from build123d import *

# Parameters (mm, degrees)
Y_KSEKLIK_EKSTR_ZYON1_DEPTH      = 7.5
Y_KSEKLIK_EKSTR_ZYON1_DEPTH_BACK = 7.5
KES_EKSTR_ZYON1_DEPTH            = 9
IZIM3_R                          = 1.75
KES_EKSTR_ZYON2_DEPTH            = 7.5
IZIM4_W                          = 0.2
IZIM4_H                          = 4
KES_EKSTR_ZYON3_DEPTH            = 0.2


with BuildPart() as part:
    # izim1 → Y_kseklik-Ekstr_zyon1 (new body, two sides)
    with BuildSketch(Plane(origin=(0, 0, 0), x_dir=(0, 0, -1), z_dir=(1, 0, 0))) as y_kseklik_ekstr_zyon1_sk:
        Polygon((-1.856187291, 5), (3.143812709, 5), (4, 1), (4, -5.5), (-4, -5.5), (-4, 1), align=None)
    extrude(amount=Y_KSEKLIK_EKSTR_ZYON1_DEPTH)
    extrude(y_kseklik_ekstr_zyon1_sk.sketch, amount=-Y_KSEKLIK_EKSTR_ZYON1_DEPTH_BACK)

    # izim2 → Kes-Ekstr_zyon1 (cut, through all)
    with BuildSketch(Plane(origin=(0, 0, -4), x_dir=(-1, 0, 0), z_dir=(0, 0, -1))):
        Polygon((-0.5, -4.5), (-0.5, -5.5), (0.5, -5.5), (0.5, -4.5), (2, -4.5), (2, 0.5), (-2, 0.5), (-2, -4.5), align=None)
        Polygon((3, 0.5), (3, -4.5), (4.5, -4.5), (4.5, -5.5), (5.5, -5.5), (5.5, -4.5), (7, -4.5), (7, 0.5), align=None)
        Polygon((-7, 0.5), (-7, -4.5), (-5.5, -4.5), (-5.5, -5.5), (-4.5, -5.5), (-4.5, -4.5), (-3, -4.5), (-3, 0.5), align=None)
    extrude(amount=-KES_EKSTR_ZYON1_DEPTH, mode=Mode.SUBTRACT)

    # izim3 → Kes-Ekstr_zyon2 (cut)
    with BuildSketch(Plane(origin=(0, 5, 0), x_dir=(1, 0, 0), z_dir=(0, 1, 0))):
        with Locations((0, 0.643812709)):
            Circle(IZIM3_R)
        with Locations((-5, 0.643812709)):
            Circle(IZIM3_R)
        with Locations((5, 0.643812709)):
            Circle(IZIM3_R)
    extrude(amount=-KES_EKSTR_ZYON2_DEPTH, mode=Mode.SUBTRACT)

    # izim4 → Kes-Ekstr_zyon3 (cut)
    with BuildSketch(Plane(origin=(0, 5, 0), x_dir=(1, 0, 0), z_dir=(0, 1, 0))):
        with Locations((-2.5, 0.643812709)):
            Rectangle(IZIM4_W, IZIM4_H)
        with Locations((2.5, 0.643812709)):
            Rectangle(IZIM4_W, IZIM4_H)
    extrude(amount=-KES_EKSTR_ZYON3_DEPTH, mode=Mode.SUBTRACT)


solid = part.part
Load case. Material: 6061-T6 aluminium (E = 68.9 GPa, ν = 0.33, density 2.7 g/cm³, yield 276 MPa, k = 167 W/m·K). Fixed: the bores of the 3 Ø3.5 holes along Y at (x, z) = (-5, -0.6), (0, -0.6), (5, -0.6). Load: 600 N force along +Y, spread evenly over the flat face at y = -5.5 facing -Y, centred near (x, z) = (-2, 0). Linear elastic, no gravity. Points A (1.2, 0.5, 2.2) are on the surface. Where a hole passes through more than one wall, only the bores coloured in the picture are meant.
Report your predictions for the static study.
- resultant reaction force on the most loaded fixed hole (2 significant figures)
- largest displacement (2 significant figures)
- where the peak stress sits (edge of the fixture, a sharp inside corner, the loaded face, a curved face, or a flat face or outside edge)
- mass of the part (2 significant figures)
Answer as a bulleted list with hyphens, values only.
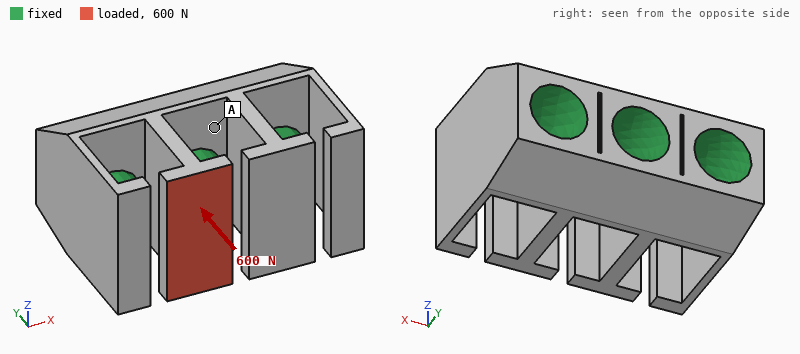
- 320 N
- 12 µm
- the loaded face
- 1.4 g
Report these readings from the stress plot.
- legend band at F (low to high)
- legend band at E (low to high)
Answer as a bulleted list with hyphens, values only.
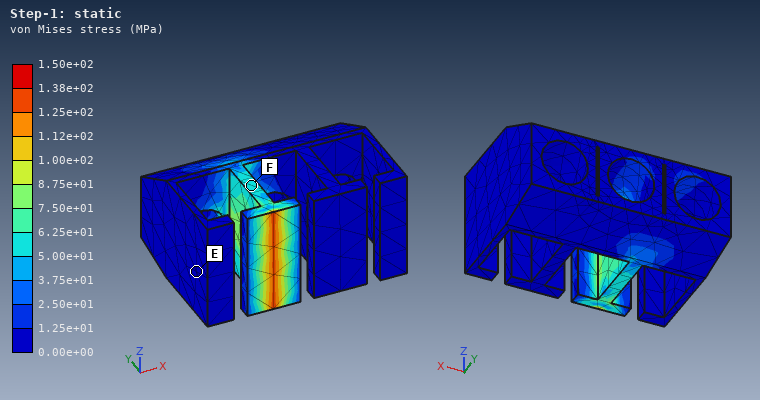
- 5.00e+01 to 6.25e+01 MPa
- 0.00e+00 to 1.25e+01 MPa
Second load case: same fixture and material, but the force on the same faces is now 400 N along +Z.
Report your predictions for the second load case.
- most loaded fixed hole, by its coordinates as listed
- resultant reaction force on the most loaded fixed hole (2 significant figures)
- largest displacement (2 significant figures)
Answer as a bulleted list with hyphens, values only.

- (0, -0.6)
- 230 N
- 40 µm
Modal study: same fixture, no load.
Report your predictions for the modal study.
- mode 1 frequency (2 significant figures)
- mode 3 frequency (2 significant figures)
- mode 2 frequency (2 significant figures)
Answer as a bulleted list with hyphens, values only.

- 6700 Hz
- 13 kHz
- 6800 Hz
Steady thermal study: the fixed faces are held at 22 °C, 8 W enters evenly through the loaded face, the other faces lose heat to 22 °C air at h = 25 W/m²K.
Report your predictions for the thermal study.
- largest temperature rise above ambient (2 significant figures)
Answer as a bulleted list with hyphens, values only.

- 38 K
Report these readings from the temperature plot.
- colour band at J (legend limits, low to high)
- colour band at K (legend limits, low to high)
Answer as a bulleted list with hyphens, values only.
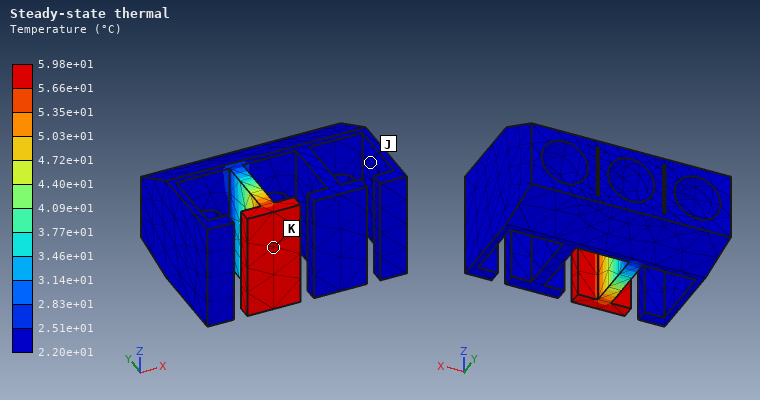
- 2.20e+01 to 2.51e+01 °C
- 5.66e+01 to 5.98e+01 °C
